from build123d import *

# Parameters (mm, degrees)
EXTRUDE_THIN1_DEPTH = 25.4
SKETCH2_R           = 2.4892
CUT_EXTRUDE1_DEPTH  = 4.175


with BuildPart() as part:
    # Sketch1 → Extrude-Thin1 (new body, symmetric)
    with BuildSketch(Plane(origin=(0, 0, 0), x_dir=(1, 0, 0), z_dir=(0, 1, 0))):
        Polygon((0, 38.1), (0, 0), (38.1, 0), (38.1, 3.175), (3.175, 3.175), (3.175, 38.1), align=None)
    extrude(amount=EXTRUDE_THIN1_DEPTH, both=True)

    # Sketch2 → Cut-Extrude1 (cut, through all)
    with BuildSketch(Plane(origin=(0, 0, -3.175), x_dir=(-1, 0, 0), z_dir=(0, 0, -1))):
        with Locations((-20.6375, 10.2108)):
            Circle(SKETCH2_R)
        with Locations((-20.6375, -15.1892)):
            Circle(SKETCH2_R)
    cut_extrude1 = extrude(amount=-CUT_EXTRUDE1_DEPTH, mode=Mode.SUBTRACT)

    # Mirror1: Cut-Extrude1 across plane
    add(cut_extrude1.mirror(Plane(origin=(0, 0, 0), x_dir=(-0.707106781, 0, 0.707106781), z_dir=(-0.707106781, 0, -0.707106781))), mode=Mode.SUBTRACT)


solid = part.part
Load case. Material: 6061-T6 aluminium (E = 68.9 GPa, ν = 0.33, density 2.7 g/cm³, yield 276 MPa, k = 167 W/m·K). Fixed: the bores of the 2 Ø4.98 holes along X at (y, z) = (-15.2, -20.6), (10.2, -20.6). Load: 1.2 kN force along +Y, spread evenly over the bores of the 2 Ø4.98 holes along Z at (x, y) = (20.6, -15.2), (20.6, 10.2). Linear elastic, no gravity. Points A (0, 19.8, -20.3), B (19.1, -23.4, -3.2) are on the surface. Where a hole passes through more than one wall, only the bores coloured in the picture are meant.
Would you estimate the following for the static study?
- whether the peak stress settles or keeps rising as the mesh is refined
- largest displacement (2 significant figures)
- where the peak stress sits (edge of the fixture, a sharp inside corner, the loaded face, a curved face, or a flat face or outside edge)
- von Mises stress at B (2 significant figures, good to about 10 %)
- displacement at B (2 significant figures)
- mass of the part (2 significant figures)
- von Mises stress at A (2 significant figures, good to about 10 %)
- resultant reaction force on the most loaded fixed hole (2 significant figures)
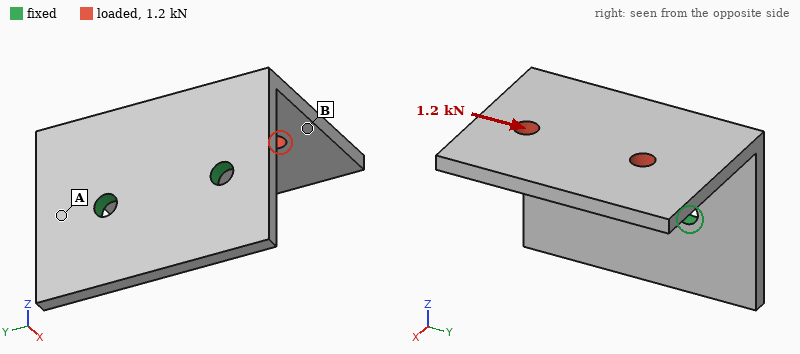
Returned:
keeps rising
0.52 mm
edge of the fixture
35 MPa
0.32 mm
31 g
100 MPa
1.2 kN
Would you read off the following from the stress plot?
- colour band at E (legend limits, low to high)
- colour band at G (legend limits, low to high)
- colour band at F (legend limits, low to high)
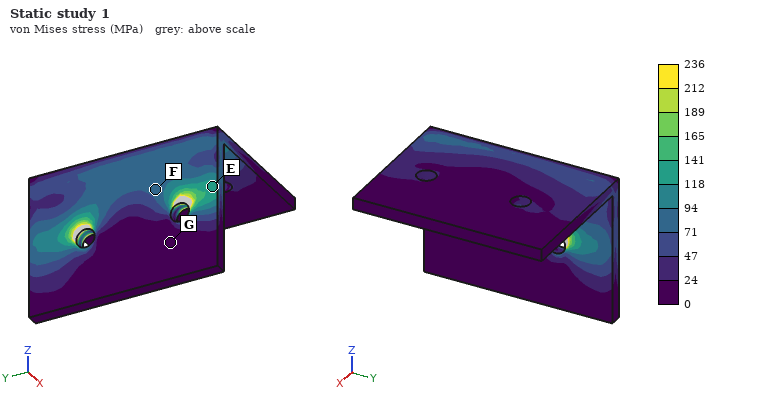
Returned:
118 to 141 MPa
0 to 24 MPa
71 to 94 MPa
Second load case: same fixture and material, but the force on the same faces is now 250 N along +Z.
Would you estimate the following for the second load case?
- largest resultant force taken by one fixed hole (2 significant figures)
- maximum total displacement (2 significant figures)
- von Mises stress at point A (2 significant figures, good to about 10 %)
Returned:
130 N
0.47 mm
25 MPa
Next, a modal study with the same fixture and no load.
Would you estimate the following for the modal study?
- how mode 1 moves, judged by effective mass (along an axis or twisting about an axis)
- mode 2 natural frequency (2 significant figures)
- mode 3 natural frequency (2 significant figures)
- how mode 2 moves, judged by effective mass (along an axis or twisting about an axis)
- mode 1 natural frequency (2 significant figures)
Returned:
along Z
2100 Hz
3500 Hz
along Y
1100 Hz
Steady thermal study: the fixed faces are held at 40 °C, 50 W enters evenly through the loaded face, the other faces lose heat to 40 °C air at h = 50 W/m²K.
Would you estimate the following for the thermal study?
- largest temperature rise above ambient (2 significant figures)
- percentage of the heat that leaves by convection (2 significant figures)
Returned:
67 K
24 %
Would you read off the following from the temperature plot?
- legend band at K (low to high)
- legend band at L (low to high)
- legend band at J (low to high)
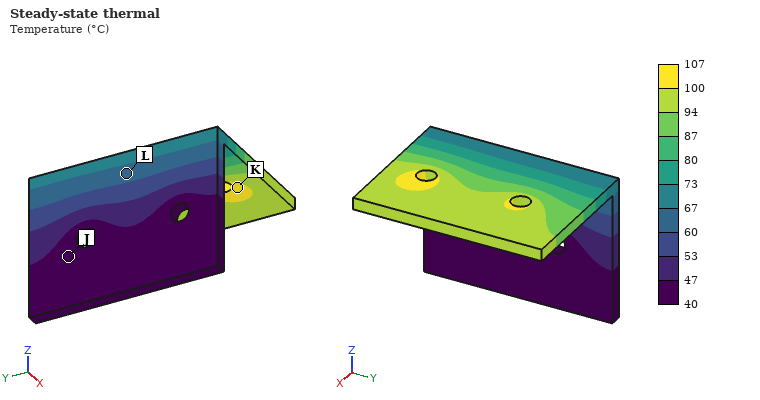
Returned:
100 to 107 °C
60 to 67 °C
40 to 47 °C
